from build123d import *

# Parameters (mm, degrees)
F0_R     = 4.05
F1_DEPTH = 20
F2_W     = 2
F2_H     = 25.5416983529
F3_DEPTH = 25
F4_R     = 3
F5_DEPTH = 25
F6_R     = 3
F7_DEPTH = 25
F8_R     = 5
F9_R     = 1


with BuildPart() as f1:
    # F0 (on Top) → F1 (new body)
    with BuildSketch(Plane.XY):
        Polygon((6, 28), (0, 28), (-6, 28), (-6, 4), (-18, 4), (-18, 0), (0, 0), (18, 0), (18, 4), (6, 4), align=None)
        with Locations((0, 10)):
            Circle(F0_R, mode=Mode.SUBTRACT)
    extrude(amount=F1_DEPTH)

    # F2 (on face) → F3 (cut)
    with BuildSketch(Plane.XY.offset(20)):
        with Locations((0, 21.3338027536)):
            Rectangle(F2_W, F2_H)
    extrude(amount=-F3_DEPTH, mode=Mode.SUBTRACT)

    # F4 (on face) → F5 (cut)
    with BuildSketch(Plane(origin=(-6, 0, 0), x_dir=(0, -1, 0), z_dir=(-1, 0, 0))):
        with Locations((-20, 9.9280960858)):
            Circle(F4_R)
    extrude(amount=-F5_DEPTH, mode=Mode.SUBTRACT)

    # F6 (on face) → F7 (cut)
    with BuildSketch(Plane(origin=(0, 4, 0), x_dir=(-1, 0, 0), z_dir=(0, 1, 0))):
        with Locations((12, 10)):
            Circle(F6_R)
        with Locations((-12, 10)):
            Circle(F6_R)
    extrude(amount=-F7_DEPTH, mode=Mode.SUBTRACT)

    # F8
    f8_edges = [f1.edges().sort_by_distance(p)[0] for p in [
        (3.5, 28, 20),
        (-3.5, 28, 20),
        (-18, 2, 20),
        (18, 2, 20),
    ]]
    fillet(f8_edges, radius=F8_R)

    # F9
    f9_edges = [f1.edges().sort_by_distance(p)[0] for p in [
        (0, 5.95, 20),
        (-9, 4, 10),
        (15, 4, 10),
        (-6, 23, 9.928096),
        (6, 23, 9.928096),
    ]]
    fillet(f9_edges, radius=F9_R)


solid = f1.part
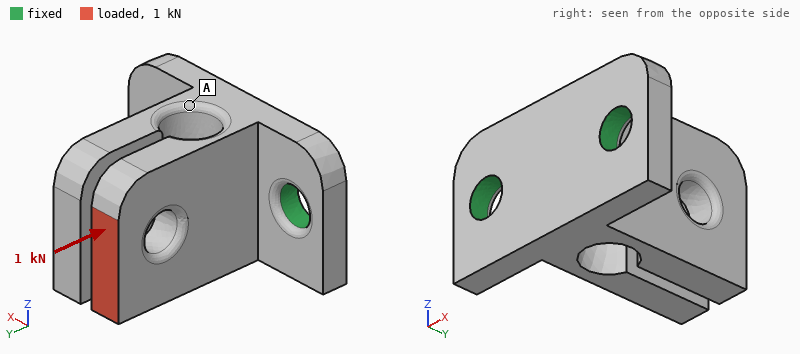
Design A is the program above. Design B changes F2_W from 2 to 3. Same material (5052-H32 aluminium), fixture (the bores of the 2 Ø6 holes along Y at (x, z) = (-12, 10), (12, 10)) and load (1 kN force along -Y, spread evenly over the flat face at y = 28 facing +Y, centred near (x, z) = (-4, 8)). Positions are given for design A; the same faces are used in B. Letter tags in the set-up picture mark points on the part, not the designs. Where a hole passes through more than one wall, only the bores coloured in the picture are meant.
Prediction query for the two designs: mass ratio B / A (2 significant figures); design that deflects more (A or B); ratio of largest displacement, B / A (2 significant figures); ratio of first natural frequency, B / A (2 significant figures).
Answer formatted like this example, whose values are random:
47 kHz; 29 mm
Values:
0.96; A; 0.81; 1.1
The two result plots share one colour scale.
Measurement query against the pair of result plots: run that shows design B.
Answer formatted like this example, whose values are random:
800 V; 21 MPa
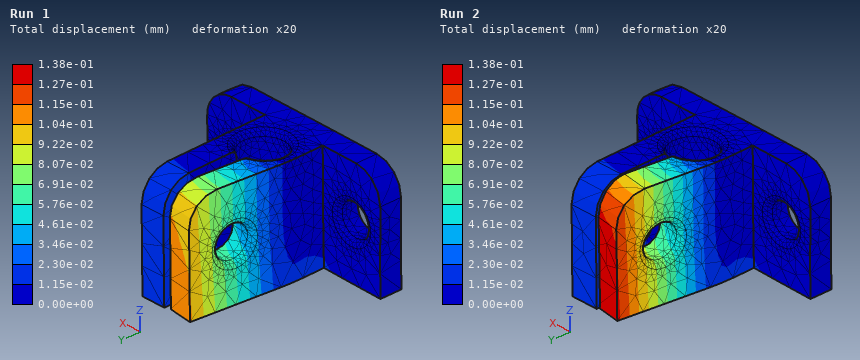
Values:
Run 1
